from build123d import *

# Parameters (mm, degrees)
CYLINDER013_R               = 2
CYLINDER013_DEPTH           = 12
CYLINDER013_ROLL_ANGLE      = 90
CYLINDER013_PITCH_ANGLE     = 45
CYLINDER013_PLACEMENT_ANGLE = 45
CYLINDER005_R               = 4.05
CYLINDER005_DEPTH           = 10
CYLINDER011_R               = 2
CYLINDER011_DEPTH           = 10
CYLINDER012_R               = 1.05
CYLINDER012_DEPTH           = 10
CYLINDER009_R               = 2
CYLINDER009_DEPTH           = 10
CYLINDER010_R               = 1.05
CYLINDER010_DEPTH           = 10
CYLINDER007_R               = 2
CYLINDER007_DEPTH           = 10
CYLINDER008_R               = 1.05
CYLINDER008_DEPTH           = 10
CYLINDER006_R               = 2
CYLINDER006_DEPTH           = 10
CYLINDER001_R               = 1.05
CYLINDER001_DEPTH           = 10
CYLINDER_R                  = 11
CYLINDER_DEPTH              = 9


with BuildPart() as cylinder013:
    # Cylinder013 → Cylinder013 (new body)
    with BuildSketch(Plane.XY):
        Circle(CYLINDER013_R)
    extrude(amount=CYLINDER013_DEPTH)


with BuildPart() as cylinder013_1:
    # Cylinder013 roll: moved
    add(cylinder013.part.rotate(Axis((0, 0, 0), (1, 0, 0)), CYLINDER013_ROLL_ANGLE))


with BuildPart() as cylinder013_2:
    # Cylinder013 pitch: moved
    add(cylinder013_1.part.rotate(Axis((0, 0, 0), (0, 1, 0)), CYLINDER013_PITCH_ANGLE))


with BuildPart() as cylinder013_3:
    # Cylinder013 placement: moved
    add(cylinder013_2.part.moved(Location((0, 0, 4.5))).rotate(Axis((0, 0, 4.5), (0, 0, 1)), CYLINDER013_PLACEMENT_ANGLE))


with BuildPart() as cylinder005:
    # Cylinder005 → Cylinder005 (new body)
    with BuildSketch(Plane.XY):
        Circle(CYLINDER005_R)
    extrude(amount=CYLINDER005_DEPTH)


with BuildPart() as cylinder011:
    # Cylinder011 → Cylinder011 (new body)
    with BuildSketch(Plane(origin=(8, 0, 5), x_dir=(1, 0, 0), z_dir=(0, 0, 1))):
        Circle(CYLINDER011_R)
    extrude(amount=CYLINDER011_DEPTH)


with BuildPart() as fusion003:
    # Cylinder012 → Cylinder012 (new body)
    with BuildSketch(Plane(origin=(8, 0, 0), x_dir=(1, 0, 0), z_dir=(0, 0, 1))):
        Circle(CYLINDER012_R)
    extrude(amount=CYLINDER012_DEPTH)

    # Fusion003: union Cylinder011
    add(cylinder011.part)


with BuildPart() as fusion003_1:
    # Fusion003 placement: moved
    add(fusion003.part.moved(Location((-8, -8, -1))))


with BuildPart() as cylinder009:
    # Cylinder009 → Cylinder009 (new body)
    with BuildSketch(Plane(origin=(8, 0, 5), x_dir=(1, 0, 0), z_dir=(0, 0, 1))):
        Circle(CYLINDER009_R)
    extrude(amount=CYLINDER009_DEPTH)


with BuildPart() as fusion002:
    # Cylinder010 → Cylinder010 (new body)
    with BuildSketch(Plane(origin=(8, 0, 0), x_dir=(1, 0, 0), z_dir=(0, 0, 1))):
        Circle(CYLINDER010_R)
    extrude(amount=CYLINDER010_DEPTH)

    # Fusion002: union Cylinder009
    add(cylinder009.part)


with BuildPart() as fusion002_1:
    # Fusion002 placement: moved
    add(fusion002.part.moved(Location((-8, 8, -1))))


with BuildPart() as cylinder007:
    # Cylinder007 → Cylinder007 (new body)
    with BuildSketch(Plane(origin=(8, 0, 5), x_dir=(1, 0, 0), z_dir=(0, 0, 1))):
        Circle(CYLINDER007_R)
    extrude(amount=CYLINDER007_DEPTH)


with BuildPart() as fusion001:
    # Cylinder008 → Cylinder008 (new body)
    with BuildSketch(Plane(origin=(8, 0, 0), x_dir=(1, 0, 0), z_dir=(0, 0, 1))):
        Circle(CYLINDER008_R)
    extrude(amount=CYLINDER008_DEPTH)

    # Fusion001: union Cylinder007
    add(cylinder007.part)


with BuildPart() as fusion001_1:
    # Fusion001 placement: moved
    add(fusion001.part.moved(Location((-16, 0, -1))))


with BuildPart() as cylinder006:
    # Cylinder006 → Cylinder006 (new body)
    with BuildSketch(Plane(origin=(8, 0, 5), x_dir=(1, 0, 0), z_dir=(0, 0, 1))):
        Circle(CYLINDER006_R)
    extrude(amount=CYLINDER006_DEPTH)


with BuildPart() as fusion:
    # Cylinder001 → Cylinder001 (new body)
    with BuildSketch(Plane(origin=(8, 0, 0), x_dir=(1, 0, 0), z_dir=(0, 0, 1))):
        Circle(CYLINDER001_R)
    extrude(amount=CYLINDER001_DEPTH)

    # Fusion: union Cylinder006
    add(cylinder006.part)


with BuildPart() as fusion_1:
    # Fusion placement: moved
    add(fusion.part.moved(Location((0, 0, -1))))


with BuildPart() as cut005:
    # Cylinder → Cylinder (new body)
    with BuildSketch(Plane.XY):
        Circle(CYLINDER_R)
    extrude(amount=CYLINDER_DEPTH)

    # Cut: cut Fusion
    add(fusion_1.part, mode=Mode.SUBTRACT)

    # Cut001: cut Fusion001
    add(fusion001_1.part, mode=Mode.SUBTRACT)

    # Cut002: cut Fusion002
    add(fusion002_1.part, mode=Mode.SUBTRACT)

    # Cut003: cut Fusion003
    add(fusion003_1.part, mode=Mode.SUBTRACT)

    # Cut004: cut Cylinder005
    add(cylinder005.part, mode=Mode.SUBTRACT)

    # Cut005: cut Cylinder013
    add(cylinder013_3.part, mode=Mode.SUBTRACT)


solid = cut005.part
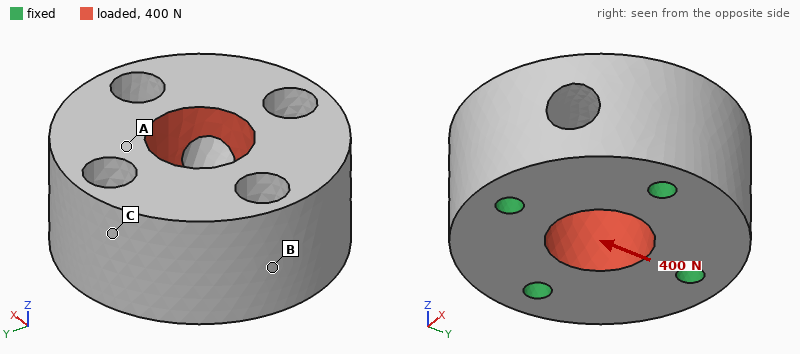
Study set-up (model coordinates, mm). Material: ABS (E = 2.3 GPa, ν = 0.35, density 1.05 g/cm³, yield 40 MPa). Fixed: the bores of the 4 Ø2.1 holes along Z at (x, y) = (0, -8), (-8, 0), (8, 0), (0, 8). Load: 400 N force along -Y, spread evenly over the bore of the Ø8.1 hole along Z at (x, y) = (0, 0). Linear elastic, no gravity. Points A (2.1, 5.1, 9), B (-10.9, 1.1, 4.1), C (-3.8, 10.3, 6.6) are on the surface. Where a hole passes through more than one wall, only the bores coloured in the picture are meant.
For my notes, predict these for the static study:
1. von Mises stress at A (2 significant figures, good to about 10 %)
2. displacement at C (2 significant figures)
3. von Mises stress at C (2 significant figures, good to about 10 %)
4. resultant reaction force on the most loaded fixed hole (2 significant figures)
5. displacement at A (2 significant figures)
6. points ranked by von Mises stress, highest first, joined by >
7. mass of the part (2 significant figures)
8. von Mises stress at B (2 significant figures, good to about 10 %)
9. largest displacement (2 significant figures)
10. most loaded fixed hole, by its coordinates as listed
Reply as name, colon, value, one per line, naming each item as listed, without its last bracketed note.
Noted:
von Mises stress at A: 4.0 MPa
displacement at C: 15 µm
von Mises stress at C: 1.9 MPa
resultant reaction force on the most loaded fixed hole: 120 N
displacement at A: 20 µm
points ranked by von Mises stress, highest first, joined by >: A > C > B
mass of the part: 2.7 g
von Mises stress at B: 1.0 MPa
largest displacement: 25 µm
most loaded fixed hole, by its coordinates as listed: (0, 8)
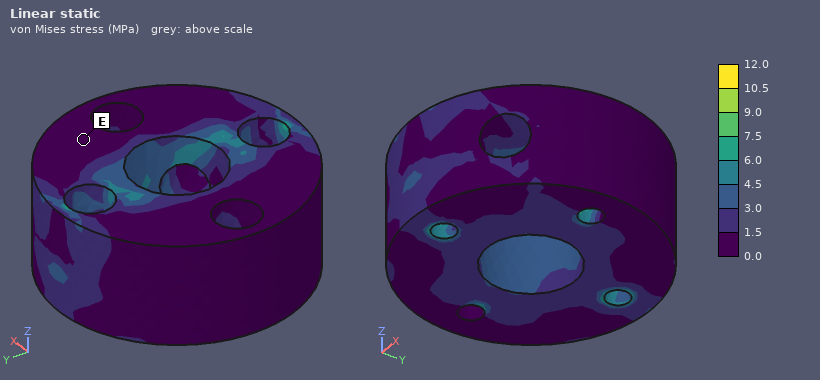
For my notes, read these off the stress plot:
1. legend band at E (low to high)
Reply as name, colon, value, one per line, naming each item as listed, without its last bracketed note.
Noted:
legend band at E: 0.0 to 1.5 MPa
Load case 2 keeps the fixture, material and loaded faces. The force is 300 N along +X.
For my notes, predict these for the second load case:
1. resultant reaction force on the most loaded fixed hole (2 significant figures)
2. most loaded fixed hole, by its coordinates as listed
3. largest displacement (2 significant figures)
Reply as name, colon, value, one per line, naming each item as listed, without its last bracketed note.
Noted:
resultant reaction force on the most loaded fixed hole: 92 N
most loaded fixed hole, by its coordinates as listed: (-8, 0)
largest displacement: 19 µm
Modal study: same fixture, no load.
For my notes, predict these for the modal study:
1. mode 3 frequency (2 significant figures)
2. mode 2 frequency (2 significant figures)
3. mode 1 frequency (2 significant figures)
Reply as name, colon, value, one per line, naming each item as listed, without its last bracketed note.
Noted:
mode 3 frequency: 17 kHz
mode 2 frequency: 16 kHz
mode 1 frequency: 16 kHz
